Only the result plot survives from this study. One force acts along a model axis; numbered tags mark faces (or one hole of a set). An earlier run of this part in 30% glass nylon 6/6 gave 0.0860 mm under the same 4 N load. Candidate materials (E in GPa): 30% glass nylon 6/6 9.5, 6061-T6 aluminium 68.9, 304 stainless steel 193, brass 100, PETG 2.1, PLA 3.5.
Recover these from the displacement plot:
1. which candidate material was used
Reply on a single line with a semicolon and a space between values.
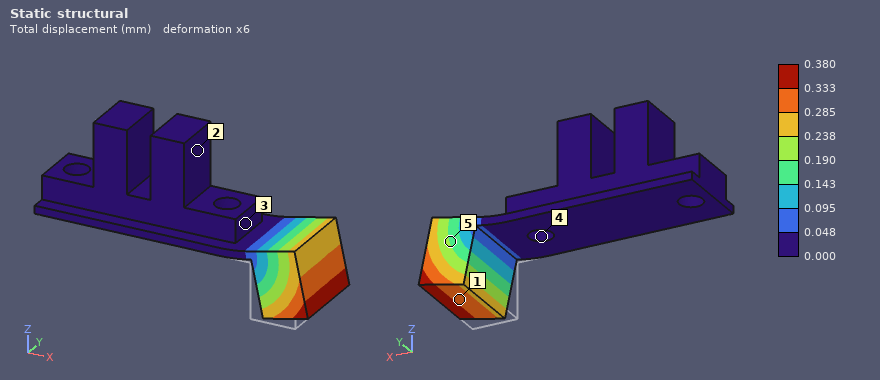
PETG
